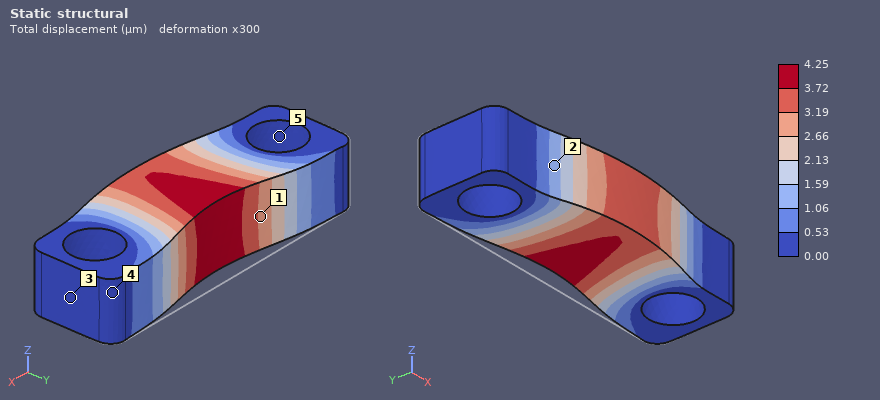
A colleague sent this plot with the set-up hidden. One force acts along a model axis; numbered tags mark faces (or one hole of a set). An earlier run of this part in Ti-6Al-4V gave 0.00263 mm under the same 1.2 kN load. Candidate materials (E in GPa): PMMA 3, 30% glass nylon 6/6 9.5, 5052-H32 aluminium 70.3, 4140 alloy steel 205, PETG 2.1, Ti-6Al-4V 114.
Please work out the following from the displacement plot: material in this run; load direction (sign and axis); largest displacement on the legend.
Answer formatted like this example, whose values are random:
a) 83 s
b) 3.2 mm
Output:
a) 5052-H32 aluminium
b) -Y
c) 4.25 µm
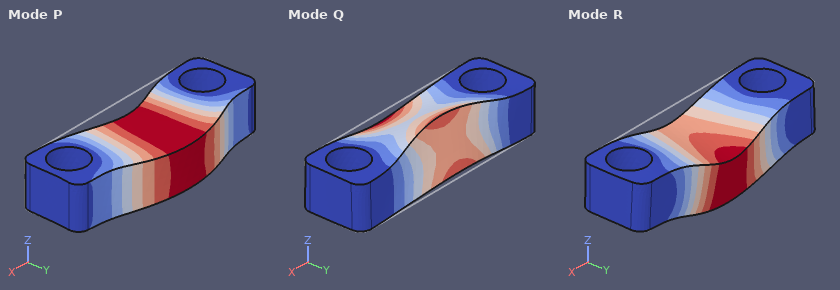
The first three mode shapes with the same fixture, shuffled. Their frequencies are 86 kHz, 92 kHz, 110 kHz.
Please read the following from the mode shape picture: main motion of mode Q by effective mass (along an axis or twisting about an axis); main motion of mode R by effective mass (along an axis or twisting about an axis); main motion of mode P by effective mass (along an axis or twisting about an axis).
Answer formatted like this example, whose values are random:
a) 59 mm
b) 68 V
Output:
a) twisting about X
b) along Z
c) along Y
